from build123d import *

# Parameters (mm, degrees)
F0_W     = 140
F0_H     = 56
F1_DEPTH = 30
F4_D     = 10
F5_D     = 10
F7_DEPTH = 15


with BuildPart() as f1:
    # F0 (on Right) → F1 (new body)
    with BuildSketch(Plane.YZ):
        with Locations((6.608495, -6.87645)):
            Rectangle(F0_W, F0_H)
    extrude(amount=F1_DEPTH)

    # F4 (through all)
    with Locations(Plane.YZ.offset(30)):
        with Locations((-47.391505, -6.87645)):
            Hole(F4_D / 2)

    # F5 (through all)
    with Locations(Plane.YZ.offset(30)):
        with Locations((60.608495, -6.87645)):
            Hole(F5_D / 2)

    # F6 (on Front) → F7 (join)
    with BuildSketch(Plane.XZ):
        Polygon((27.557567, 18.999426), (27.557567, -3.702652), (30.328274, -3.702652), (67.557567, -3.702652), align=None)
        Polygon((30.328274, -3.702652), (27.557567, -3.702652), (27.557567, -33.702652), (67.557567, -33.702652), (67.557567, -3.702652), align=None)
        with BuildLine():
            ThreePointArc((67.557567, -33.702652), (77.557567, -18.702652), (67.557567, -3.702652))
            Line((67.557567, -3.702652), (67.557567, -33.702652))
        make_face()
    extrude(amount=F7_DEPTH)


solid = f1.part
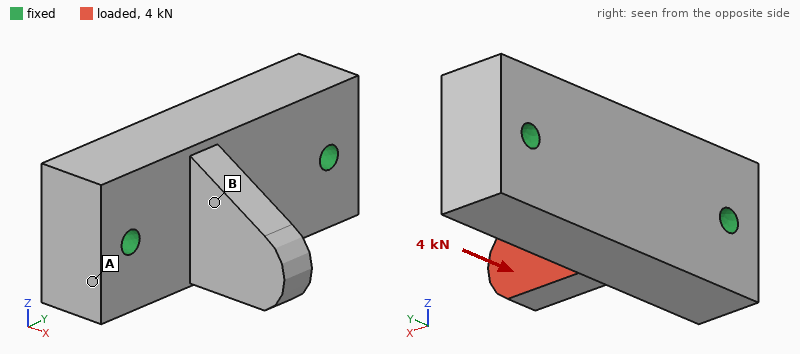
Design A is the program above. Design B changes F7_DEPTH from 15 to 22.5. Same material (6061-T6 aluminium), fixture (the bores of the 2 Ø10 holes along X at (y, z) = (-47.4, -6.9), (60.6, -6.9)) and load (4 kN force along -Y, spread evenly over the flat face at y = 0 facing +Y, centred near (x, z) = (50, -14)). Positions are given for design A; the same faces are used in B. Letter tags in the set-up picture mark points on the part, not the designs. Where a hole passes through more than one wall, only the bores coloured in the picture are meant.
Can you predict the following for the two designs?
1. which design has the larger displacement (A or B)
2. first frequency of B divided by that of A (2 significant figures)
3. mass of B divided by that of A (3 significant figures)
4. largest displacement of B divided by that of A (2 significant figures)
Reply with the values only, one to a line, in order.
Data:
A
1.0
1.05
0.43
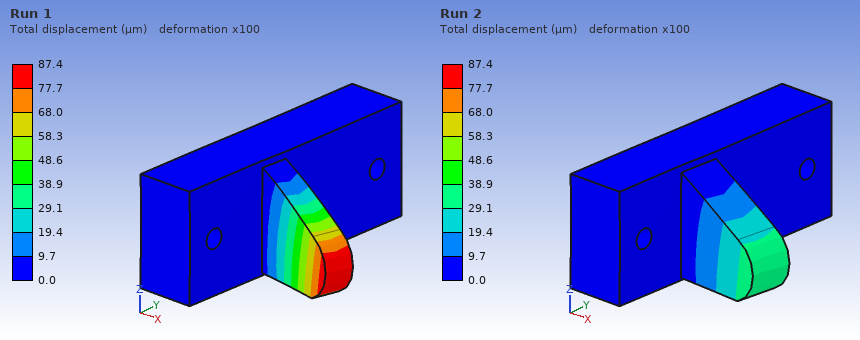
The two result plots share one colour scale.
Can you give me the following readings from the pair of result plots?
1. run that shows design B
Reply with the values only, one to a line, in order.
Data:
Run 2
